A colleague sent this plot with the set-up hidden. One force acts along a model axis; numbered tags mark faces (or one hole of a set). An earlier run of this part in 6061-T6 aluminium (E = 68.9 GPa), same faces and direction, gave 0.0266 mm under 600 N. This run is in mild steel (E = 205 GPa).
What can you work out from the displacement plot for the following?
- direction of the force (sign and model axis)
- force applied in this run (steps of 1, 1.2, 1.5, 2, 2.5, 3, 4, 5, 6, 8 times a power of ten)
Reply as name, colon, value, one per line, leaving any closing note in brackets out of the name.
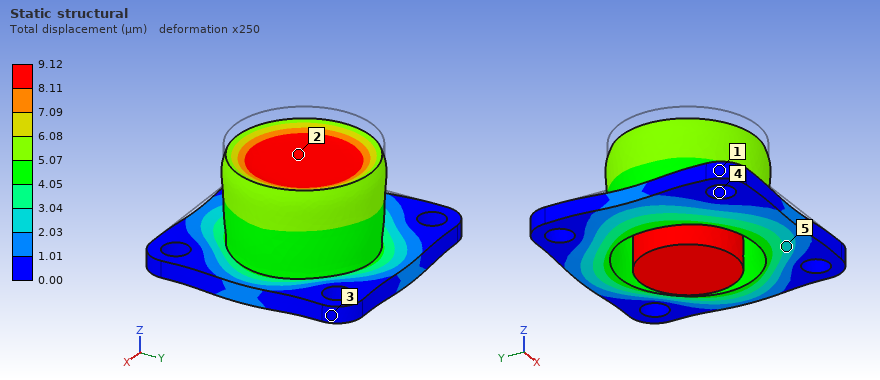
direction of the force: -Z
force applied in this run: 600 N
